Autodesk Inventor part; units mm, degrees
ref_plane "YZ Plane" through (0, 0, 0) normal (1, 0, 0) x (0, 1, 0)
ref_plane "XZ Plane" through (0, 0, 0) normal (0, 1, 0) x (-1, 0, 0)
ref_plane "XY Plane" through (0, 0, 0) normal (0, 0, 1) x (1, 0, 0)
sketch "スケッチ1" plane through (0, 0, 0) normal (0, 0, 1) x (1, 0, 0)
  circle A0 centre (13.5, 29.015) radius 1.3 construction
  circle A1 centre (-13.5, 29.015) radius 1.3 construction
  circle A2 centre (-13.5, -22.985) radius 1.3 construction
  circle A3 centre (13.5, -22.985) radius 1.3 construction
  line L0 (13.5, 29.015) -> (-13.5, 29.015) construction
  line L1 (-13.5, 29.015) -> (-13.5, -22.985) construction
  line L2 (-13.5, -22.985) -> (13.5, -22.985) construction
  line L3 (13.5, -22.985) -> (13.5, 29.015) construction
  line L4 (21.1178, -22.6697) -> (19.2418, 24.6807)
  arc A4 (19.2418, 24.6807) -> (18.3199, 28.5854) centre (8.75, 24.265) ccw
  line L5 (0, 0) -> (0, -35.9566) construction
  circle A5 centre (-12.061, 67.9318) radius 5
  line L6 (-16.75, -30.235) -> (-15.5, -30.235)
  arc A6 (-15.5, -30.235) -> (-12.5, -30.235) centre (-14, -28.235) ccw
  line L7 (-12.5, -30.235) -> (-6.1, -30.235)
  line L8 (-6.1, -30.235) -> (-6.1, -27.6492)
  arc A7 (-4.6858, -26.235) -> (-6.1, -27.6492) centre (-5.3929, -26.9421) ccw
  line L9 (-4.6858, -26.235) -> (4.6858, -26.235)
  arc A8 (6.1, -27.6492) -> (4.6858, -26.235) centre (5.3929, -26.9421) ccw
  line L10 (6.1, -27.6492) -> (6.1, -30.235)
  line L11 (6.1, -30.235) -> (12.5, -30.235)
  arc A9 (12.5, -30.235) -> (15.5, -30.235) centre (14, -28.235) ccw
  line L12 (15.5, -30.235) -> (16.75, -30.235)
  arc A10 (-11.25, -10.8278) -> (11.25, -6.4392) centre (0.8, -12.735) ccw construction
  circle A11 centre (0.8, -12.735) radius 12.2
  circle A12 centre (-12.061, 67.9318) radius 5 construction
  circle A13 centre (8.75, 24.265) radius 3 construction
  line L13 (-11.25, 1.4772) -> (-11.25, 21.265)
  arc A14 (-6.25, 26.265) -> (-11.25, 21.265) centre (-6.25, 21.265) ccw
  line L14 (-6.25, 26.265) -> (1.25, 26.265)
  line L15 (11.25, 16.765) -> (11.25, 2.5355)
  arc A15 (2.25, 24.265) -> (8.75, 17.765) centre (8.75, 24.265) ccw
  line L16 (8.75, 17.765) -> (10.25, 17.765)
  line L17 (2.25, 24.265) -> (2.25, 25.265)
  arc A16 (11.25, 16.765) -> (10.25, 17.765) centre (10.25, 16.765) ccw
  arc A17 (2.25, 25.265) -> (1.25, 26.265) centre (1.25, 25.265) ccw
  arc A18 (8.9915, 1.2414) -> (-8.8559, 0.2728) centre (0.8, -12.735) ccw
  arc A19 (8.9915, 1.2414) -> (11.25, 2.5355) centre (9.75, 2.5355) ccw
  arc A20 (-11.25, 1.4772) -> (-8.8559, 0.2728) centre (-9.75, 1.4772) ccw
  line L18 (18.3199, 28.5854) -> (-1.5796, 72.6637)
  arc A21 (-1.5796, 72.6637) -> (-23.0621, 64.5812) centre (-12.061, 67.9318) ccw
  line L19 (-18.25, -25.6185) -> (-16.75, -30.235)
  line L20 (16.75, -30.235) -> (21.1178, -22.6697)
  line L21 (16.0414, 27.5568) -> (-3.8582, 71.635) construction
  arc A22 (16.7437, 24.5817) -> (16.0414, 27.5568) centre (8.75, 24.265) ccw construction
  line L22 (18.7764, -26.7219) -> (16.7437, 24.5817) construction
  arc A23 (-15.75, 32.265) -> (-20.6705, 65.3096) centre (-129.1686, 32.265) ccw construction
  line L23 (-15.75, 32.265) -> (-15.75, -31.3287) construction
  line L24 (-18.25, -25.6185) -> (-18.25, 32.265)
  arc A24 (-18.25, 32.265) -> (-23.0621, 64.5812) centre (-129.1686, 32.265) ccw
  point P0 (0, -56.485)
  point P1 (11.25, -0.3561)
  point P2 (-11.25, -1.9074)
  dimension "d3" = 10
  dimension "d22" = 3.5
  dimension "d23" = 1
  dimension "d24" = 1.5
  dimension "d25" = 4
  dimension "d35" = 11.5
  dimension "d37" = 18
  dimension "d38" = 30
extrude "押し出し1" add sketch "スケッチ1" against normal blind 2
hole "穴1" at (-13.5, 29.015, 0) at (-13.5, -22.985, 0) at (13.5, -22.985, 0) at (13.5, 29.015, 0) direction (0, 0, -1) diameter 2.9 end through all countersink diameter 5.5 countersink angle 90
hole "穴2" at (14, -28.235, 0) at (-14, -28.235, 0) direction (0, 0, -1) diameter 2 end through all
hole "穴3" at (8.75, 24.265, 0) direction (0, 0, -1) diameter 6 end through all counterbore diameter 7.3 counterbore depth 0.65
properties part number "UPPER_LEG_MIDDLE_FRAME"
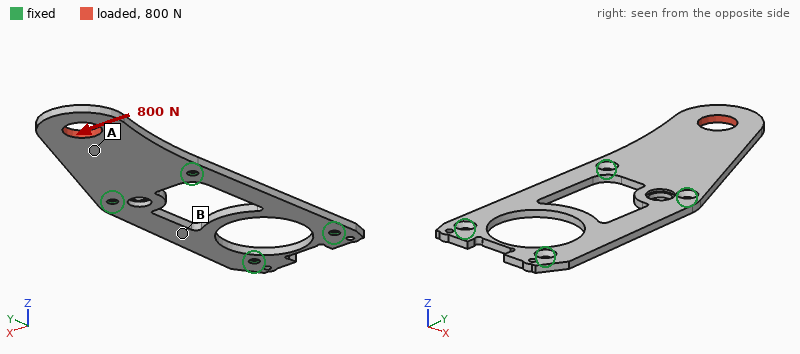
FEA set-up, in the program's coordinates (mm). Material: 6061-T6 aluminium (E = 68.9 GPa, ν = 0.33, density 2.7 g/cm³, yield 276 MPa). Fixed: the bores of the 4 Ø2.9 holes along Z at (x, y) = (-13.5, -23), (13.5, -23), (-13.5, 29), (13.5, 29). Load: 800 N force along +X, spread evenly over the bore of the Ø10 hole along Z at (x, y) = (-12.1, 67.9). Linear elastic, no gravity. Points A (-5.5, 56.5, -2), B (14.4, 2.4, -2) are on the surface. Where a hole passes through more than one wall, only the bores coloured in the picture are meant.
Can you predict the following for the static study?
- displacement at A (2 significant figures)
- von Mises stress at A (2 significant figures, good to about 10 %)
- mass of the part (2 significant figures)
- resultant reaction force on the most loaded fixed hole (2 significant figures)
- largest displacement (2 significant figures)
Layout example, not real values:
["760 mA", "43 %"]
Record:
["0.052 mm", "38 MPa", "13 g", "1.2 kN", "0.13 mm"]
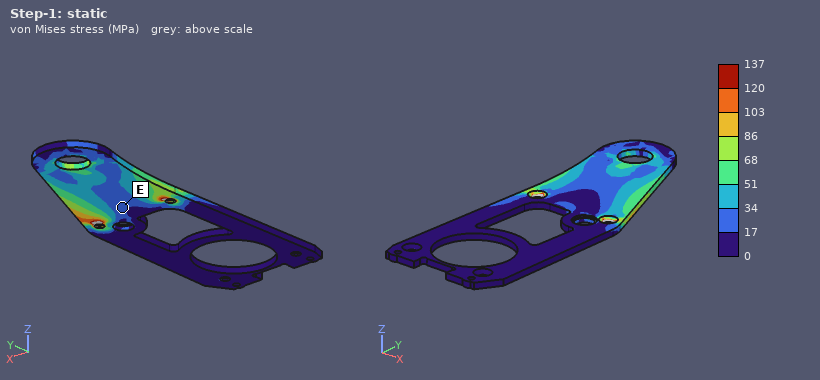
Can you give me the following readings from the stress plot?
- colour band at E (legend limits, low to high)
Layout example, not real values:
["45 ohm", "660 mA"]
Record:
["17 to 34 MPa"]
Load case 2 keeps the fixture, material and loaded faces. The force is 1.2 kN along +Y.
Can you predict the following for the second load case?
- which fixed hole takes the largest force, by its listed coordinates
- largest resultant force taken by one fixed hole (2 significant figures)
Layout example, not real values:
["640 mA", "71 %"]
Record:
["(-13.5, 29)", "1.0 kN"]
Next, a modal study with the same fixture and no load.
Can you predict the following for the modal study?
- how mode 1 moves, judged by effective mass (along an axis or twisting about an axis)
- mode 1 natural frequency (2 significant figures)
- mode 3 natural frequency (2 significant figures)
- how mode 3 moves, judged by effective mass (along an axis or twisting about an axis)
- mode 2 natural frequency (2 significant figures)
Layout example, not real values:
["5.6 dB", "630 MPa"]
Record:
["along Z", "710 Hz", "3200 Hz", "along Z", "3000 Hz"]
